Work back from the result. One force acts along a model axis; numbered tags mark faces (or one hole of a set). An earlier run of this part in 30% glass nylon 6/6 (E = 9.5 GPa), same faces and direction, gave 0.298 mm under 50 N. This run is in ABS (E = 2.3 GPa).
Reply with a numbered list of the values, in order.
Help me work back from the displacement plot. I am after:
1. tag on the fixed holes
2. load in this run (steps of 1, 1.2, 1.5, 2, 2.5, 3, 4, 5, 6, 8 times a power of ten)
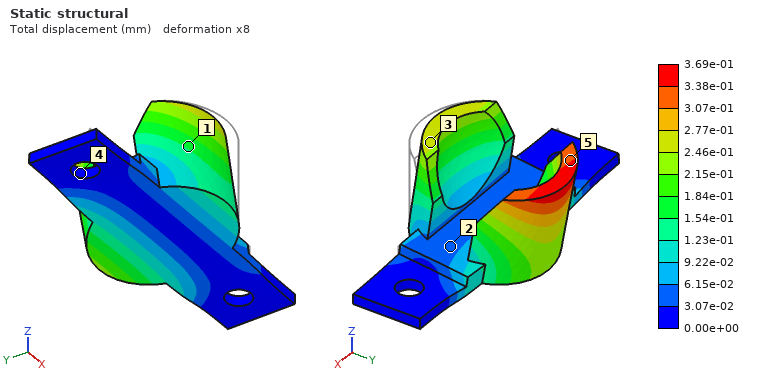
1. 4
2. 15 N
